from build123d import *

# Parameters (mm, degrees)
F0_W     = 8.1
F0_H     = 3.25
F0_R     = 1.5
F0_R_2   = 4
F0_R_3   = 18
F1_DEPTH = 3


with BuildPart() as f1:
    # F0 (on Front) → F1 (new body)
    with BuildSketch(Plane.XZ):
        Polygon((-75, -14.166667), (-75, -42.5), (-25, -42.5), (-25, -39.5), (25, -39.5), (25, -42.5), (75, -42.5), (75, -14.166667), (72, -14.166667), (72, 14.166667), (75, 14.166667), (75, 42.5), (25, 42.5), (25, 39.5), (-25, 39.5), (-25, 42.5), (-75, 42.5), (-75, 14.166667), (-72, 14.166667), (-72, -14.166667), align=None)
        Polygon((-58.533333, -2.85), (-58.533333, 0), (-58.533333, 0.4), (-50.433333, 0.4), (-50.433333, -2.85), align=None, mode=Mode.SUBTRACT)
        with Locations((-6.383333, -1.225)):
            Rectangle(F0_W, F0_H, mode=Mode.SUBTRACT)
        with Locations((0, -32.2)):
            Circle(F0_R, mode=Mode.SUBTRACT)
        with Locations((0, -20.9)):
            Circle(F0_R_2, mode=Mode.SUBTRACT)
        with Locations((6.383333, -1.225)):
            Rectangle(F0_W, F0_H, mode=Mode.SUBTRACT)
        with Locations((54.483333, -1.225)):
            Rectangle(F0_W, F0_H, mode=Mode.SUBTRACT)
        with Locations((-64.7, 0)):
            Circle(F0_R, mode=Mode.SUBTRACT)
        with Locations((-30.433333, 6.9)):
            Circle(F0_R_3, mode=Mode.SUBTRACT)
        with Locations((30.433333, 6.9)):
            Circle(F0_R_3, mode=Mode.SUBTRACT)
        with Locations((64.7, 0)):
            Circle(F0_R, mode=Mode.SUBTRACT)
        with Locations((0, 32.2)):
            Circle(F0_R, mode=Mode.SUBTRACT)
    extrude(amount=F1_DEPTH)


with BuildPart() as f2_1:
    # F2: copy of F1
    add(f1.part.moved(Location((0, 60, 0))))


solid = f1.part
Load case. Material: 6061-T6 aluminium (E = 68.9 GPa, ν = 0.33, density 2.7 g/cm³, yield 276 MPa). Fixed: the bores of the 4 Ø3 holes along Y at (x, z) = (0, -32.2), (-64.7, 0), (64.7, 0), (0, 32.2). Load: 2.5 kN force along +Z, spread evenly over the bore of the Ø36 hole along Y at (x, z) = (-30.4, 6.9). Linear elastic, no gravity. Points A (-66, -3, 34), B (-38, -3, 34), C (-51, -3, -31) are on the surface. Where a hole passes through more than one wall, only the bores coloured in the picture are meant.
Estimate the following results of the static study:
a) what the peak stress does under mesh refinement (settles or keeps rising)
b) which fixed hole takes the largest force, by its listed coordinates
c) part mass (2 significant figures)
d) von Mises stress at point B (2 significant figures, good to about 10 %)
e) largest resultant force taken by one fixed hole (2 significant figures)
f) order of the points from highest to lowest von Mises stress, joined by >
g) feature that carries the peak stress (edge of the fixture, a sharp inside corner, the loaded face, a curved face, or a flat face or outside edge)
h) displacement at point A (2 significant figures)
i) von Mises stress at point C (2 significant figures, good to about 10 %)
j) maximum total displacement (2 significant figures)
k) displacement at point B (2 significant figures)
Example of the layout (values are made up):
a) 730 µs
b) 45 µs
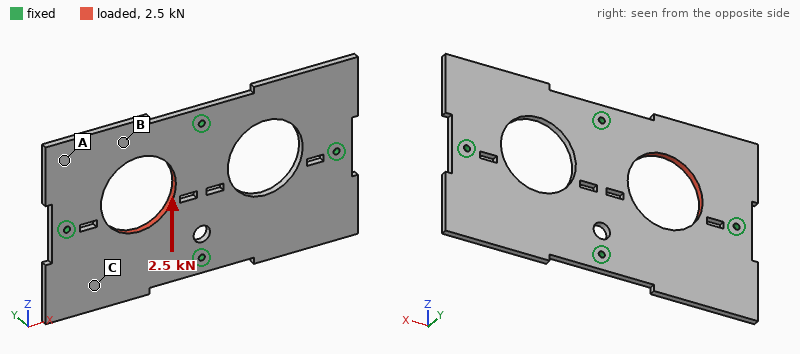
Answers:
a) keeps rising
b) (-64.7, 0)
c) 81 g
d) 10 MPa
e) 1.1 kN
f) B > C > A
g) edge of the fixture
h) 5.9 µm
i) 5.6 MPa
j) 14 µm
k) 13 µm
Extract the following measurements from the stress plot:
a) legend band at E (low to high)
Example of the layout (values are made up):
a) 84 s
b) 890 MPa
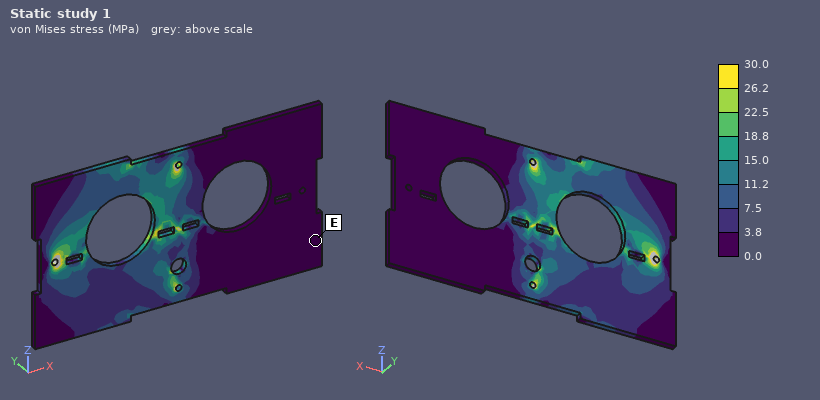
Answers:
a) 0.0 to 3.8 MPa
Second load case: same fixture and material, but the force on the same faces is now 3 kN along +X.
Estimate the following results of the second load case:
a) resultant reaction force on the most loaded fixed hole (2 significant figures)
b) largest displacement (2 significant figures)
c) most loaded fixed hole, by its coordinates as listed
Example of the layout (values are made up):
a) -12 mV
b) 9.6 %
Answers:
a) 1.2 kN
b) 12 µm
c) (0, 32.2)
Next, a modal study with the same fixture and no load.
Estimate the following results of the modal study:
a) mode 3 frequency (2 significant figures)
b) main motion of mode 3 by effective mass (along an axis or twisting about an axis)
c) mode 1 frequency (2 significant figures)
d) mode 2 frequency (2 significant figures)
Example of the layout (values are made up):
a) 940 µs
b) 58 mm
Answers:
a) 1500 Hz
b) twisting about Z
c) 1400 Hz
d) 1400 Hz
